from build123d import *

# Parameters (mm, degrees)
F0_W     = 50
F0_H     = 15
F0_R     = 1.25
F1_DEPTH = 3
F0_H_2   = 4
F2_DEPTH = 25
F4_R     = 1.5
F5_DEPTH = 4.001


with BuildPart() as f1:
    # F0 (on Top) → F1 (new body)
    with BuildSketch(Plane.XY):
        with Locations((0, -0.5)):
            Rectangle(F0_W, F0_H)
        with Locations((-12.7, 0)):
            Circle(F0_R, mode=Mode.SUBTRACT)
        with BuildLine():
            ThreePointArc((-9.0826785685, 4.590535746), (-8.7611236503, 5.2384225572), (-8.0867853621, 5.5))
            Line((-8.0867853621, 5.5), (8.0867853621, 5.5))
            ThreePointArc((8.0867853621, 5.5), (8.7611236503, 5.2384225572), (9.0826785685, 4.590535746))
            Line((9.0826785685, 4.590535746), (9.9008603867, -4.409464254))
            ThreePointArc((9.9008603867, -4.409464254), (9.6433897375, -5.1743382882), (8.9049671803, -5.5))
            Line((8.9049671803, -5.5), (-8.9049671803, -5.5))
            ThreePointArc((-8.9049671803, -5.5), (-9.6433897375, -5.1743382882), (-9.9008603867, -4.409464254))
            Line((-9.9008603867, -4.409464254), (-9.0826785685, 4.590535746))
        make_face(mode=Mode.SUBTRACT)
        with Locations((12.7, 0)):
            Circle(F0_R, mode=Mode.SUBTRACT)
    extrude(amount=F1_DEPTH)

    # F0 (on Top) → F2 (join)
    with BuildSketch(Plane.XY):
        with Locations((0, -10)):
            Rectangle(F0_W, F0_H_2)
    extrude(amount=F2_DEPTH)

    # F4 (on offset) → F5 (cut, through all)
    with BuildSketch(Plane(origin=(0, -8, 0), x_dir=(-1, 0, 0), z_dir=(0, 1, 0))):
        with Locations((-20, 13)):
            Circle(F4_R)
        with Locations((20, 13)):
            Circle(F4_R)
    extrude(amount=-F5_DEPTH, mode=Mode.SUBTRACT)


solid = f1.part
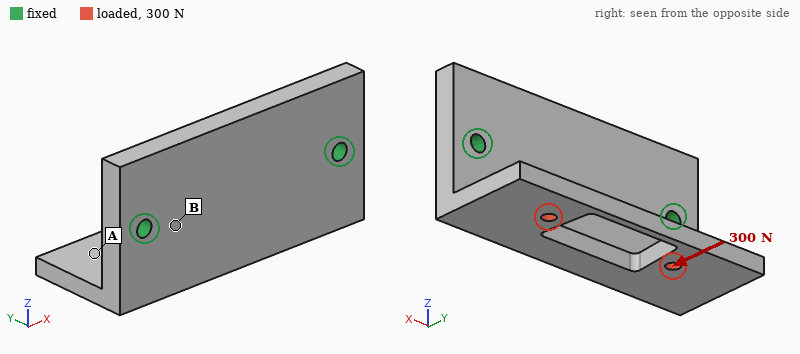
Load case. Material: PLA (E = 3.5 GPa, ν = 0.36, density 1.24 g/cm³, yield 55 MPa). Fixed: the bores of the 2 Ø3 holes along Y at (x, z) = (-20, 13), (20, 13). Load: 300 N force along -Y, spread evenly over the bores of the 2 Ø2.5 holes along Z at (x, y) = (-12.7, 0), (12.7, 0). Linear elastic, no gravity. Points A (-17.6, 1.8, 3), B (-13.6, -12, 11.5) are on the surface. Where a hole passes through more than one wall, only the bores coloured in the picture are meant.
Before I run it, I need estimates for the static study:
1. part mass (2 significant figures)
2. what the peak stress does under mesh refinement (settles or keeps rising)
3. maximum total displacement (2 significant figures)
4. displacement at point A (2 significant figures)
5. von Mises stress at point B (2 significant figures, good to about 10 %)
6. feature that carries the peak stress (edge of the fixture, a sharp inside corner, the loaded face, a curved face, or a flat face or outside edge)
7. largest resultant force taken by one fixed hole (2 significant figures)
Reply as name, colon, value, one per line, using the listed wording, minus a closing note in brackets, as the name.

part mass: 8.1 g
what the peak stress does under mesh refinement: keeps rising
maximum total displacement: 0.68 mm
displacement at point A: 0.47 mm
von Mises stress at point B: 14 MPa
feature that carries the peak stress: edge of the fixture
largest resultant force taken by one fixed hole: 150 N
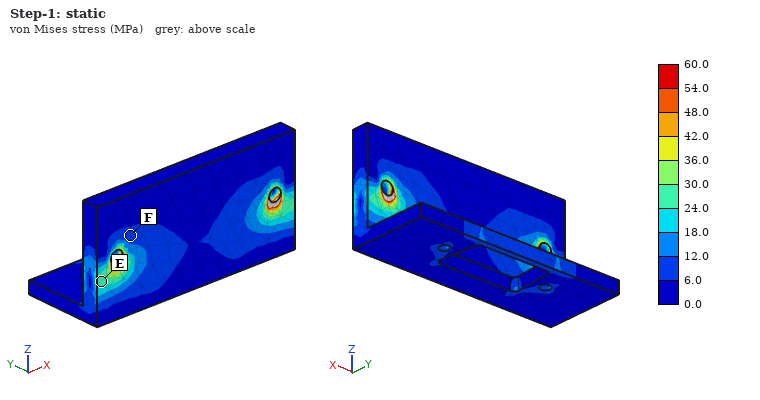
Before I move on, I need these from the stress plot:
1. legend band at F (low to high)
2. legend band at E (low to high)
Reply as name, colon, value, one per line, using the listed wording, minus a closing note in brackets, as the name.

legend band at F: 6.0 to 12.0 MPa
legend band at E: 24.0 to 30.0 MPa
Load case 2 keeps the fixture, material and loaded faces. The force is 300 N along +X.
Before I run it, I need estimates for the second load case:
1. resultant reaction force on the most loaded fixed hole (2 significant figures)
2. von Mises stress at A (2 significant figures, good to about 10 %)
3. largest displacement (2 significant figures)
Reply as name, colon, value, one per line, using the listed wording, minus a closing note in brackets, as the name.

resultant reaction force on the most loaded fixed hole: 180 N
von Mises stress at A: 4.7 MPa
largest displacement: 0.34 mm
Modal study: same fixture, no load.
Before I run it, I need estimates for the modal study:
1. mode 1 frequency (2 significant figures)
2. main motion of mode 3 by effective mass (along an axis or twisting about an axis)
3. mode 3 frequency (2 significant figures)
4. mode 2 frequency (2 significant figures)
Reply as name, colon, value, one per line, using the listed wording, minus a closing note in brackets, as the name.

mode 1 frequency: 1800 Hz
main motion of mode 3 by effective mass: along Y
mode 3 frequency: 3600 Hz
mode 2 frequency: 2300 Hz
